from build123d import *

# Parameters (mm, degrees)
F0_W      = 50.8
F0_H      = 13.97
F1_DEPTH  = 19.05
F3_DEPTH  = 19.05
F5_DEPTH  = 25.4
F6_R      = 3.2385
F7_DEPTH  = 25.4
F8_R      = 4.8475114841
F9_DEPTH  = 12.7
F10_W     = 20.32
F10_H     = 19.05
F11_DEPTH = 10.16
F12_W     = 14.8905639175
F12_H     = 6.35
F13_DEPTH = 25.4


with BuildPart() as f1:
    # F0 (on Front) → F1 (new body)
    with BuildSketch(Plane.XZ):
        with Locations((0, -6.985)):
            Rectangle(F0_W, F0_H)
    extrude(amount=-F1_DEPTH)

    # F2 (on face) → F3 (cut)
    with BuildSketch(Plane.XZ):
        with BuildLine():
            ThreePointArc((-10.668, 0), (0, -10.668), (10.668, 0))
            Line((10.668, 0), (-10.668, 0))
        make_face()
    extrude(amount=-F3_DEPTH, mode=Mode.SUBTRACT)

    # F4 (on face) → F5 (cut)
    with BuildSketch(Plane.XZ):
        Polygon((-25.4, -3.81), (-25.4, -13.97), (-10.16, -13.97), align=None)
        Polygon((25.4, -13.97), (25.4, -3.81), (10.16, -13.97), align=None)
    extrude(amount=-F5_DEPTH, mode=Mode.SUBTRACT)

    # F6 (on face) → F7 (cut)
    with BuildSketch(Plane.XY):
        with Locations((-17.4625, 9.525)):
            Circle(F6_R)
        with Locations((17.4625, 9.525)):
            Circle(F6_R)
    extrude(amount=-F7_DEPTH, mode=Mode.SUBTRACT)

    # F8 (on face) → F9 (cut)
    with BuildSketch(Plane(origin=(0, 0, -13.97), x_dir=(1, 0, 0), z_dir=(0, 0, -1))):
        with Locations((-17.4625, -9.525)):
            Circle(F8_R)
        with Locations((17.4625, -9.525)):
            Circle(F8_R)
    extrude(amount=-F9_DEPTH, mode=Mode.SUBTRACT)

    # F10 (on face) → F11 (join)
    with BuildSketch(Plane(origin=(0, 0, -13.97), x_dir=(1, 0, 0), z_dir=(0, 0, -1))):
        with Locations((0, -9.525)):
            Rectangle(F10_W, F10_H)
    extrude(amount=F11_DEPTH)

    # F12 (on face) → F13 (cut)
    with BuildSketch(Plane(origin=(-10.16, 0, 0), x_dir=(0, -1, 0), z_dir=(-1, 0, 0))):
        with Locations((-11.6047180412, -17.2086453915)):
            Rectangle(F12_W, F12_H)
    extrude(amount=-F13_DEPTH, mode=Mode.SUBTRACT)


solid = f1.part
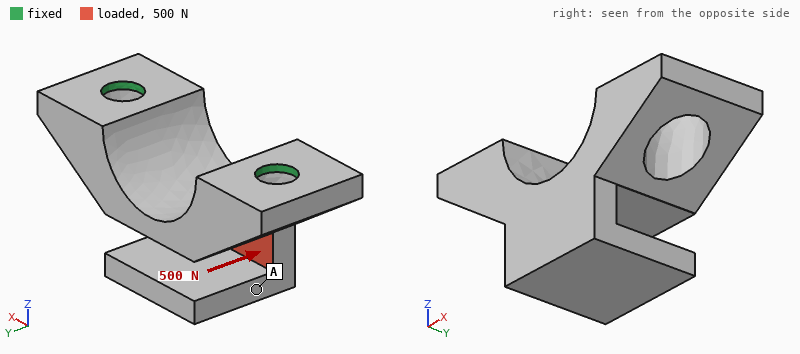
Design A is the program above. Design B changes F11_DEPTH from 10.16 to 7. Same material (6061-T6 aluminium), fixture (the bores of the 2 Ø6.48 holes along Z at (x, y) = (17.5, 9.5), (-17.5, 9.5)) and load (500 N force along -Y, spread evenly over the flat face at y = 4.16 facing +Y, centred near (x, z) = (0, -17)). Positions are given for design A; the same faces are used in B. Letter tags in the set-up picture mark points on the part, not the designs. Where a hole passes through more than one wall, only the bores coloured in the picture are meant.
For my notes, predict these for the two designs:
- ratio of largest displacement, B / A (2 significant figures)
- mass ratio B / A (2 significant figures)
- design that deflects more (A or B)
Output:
0.88
0.85
A
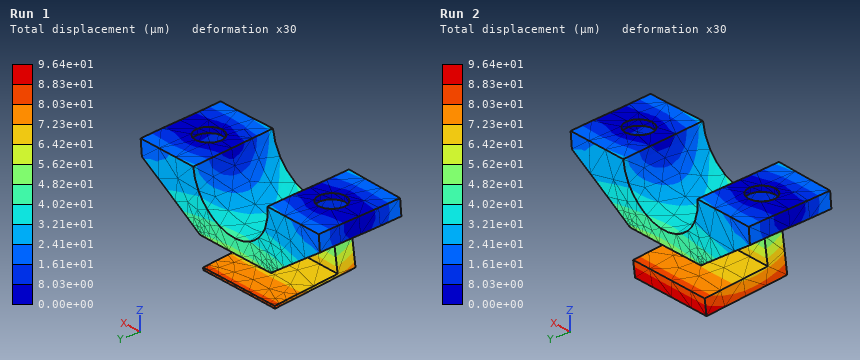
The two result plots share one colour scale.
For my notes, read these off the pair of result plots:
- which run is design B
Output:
Run 1
